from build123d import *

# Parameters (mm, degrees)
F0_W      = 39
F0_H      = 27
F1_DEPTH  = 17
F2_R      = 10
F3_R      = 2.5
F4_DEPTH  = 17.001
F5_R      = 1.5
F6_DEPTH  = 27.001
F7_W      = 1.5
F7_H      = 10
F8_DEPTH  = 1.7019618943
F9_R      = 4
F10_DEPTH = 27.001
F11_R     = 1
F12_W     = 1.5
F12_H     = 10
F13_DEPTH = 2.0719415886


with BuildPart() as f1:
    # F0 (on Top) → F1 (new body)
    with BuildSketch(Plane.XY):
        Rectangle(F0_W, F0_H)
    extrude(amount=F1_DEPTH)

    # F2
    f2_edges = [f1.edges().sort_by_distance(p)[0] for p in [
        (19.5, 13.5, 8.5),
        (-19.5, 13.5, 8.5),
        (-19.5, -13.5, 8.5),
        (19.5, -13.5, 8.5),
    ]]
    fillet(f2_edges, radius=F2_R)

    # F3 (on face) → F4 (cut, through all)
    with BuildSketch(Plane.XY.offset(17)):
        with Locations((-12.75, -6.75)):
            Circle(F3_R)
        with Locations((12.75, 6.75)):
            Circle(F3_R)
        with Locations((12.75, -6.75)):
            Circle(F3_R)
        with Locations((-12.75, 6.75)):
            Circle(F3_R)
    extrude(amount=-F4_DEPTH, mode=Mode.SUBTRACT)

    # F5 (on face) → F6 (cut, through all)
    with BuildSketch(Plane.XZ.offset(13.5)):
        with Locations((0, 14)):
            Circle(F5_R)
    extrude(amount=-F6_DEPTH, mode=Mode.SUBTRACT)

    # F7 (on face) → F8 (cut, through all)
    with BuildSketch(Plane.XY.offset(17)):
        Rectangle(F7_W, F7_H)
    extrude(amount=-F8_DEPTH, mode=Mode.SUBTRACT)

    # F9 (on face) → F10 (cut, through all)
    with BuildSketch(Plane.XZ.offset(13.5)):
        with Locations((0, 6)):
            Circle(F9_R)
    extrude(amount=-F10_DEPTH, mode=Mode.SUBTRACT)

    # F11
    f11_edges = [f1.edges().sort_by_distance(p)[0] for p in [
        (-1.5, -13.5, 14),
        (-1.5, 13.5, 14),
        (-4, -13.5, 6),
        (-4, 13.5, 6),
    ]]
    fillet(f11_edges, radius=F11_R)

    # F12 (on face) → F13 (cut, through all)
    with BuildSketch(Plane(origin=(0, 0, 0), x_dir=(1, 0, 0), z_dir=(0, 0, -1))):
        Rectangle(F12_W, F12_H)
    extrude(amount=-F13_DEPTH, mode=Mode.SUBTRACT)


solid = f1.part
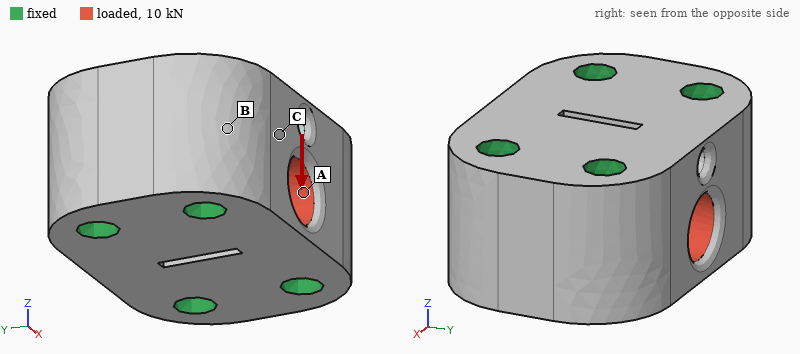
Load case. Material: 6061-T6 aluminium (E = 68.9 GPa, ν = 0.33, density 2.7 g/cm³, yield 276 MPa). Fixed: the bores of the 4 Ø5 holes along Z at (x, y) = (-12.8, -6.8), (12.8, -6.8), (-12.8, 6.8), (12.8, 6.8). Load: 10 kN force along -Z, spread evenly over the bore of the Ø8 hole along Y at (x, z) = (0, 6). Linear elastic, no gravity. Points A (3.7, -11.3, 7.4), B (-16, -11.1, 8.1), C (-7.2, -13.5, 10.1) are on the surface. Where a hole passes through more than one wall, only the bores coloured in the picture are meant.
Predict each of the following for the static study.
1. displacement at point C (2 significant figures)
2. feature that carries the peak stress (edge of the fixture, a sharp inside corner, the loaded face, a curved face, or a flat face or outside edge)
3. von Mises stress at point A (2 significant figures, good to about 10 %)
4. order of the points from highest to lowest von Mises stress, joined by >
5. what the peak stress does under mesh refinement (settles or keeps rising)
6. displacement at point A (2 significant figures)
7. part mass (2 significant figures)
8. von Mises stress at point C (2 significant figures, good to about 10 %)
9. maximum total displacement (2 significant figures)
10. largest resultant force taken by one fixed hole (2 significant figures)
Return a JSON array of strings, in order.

["2.5 µm", "a sharp inside corner", "29 MPa", "A > C > B", "keeps rising", "4.4 µm", "36 g", "19 MPa", "12 µm", "2.5 kN"]
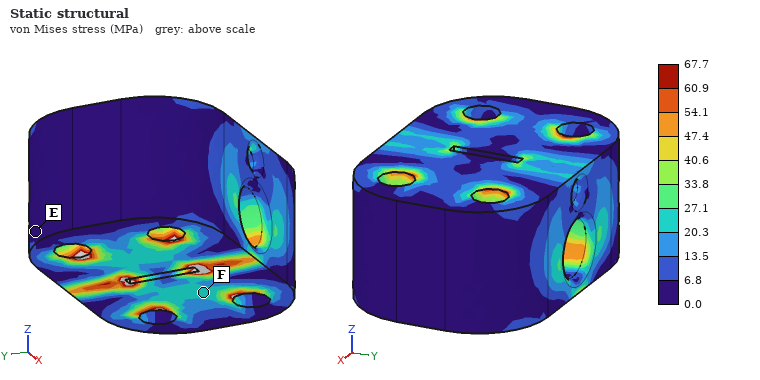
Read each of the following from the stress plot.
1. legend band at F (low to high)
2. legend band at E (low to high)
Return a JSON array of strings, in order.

["20.3 to 27.1 MPa", "0.0 to 6.8 MPa"]
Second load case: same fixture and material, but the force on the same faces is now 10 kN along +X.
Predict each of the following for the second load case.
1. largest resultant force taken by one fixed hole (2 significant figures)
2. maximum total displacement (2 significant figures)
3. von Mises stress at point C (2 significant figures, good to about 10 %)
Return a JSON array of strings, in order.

["2.5 kN", "2.9 µm", "6.6 MPa"]
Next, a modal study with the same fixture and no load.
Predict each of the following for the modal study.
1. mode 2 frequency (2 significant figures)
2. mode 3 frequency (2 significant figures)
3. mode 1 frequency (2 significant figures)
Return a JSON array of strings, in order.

["65 kHz", "68 kHz", "64 kHz"]
